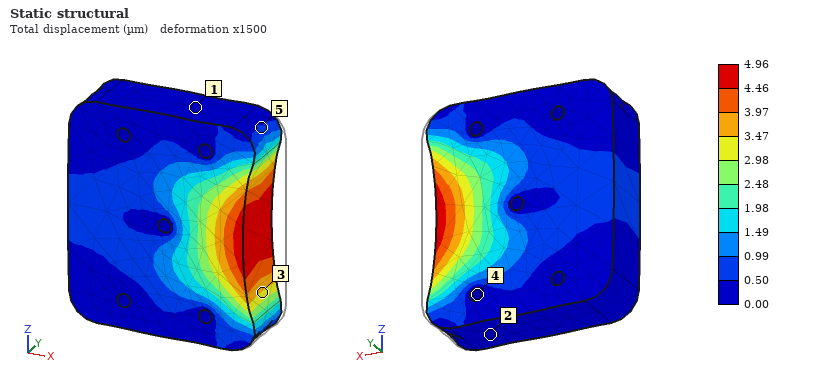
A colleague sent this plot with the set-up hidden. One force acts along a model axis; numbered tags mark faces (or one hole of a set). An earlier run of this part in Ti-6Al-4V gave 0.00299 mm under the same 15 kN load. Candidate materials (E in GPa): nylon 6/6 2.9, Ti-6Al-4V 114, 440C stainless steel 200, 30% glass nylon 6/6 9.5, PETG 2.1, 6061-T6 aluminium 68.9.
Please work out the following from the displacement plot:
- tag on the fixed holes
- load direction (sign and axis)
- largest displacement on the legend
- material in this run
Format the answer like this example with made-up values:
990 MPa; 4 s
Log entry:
4; -X; 4.96 µm; 6061-T6 aluminium
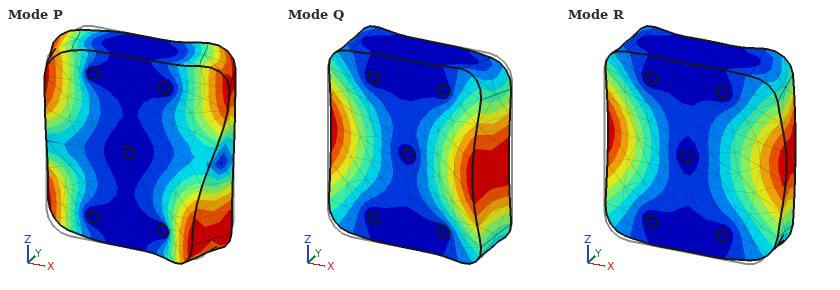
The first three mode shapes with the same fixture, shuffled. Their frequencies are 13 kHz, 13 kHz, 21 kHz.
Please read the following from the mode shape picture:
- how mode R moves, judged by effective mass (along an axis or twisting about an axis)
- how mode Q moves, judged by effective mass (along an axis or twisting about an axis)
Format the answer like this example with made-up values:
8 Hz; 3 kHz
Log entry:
along Y; twisting about Z
